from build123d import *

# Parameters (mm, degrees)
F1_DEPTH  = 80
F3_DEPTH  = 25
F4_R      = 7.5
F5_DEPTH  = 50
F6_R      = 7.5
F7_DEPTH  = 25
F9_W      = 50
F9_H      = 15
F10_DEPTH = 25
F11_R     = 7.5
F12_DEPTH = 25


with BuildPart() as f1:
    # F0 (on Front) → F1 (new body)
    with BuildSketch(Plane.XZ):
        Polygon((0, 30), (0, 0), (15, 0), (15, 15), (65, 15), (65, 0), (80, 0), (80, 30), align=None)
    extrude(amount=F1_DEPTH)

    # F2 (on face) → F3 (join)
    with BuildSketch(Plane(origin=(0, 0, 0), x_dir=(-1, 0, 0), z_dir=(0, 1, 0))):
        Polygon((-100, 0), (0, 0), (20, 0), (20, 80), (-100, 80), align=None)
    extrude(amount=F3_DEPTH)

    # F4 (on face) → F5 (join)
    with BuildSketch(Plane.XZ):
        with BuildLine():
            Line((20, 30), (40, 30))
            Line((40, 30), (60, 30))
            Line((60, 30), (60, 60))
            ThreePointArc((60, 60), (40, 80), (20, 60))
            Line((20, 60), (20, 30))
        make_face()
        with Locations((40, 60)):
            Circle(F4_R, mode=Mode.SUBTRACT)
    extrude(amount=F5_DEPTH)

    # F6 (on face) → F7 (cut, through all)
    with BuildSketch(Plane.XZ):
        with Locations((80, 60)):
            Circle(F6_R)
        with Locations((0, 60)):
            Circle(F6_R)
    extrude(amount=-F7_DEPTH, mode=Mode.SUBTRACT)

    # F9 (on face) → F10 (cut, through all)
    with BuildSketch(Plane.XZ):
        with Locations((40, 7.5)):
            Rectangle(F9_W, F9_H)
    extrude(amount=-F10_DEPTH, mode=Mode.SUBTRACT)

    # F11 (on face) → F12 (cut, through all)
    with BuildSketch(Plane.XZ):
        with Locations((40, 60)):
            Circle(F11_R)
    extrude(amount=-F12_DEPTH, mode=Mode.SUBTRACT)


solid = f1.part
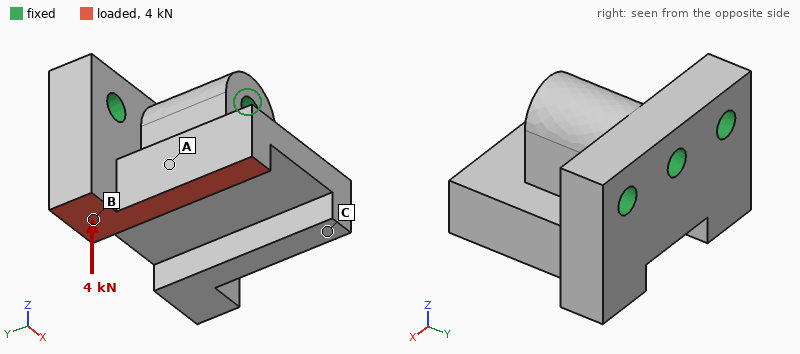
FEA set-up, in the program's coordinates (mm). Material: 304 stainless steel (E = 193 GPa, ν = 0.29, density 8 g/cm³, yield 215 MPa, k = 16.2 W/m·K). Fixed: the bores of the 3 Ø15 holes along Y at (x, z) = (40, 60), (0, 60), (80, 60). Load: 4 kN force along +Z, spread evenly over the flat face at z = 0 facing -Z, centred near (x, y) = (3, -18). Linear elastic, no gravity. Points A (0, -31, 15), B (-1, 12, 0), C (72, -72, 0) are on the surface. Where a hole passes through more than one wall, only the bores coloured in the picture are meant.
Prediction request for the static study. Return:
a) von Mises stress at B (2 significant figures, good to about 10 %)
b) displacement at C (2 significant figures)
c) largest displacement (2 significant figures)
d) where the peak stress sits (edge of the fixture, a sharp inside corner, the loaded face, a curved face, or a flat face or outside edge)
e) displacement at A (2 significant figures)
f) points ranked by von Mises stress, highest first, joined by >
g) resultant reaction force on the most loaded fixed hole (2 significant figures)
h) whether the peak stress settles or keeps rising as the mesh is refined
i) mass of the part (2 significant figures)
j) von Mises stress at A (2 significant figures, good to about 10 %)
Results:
2.3 MPa
1.8 µm
9.2 µm
a sharp inside corner
3.6 µm
A > B > C
2.5 kN
keeps rising
3.4 kg
4.6 MPa
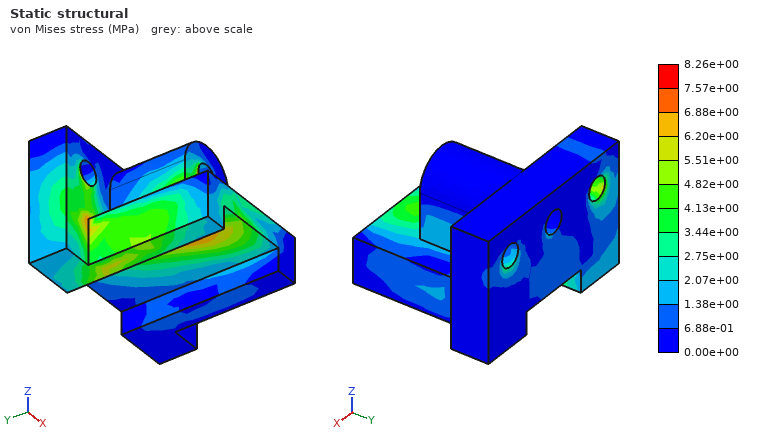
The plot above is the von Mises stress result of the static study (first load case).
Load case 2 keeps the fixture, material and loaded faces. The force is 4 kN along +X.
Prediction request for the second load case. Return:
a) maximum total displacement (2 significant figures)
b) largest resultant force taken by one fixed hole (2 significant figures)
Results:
13 µm
2.9 kN
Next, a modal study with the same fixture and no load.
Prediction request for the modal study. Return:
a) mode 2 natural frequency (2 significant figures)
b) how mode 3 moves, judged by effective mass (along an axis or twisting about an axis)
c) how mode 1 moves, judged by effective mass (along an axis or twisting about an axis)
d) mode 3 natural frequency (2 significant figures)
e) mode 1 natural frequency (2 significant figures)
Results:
5600 Hz
twisting about Z
along X
6500 Hz
4600 Hz
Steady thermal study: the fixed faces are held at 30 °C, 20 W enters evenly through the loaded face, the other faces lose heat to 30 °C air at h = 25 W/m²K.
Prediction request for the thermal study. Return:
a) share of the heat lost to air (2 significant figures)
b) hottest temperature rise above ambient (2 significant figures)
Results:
32 %
27 K
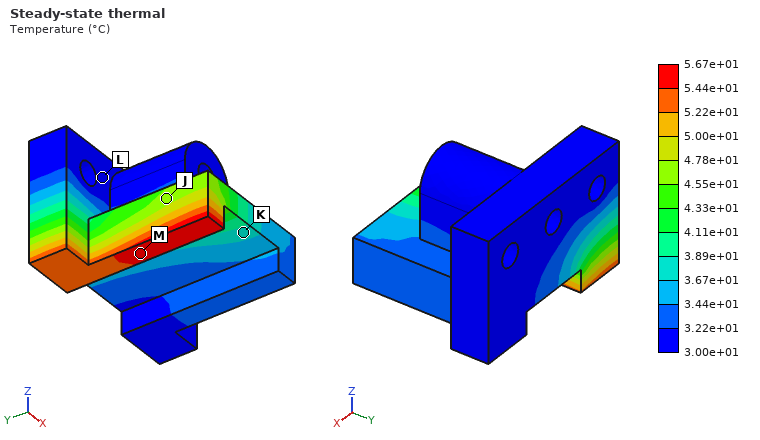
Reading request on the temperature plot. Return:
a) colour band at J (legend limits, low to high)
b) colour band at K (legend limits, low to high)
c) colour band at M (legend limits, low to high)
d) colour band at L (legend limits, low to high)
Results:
4.55e+01 to 4.78e+01 °C
3.67e+01 to 3.89e+01 °C
5.44e+01 to 5.67e+01 °C
3.00e+01 to 3.22e+01 °C
